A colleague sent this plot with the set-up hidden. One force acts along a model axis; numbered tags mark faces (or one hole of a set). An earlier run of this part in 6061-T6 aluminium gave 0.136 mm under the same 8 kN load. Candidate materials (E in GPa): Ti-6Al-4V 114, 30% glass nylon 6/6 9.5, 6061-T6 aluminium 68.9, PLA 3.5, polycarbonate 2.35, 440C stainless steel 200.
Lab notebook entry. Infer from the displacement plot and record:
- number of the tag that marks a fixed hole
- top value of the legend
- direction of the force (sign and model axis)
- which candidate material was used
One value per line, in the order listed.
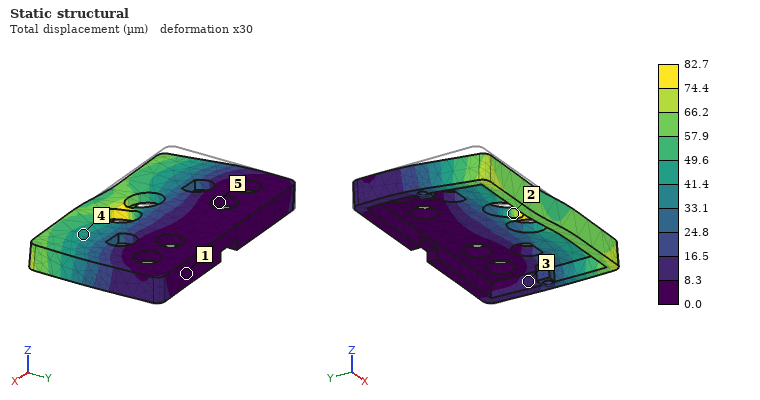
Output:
5
82.7 µm
+X
Ti-6Al-4V
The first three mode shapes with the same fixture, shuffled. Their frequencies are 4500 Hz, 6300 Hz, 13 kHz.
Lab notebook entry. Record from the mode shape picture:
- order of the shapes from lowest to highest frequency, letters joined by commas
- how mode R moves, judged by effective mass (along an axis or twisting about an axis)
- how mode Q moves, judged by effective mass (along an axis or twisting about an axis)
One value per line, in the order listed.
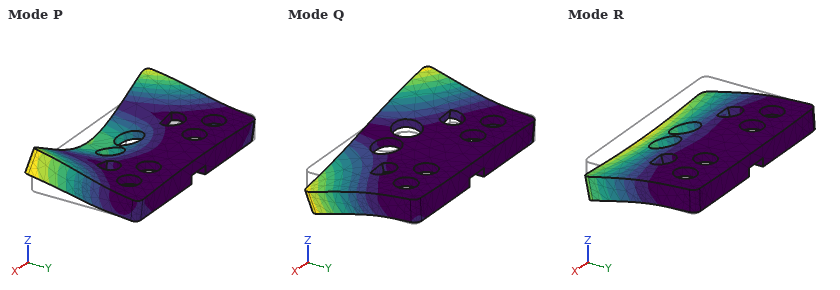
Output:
R, Q, P
along Z
twisting about Y
